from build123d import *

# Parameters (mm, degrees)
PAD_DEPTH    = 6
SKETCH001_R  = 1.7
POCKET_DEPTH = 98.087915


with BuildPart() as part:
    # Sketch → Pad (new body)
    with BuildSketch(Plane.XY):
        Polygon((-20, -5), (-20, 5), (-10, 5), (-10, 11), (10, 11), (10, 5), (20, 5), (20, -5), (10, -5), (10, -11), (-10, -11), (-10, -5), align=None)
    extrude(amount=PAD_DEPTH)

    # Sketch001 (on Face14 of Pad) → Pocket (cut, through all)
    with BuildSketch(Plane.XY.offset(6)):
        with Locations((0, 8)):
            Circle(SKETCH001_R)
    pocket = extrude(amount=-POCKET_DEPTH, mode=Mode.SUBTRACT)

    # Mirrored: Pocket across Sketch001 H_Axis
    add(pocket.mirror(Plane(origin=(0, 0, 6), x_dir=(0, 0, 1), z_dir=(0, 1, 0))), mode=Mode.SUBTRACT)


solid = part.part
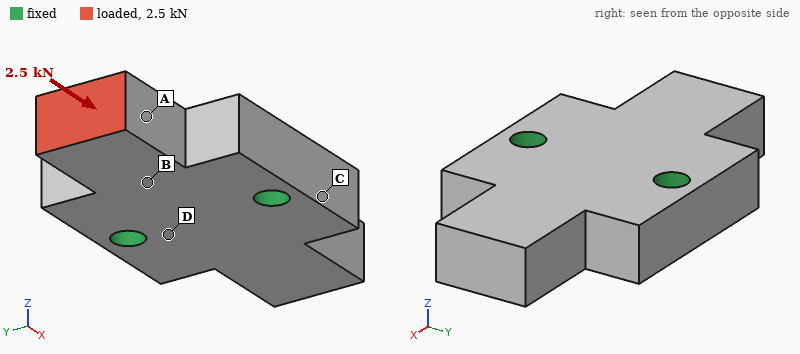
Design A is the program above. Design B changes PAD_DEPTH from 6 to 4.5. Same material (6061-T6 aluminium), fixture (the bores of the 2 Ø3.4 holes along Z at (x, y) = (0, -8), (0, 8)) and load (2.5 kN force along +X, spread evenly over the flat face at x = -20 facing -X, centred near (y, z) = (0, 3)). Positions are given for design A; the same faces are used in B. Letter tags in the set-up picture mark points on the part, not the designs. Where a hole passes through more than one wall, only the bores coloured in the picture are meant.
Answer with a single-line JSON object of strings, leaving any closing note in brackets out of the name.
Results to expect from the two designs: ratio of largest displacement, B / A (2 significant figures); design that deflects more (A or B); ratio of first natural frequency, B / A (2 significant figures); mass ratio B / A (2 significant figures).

{"ratio of largest displacement, B / A": "1.3", "design that deflects more": "B", "ratio of first natural frequency, B / A": "0.80", "mass ratio B / A": "0.75"}
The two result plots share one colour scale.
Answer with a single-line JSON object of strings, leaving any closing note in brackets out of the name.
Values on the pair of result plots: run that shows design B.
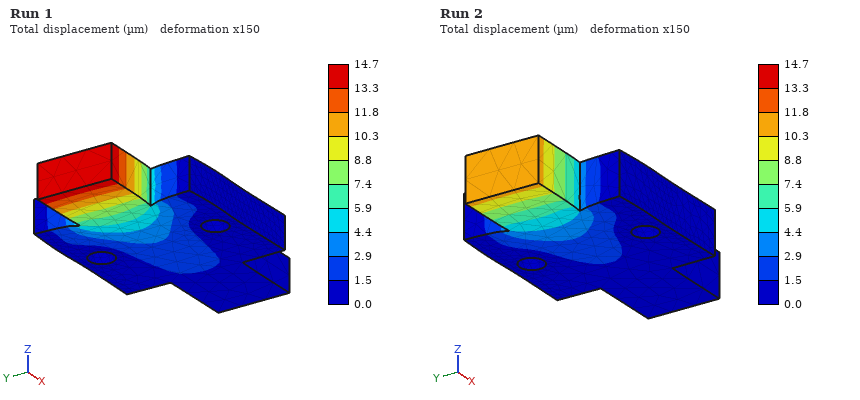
{"run that shows design B": "Run 1"}
